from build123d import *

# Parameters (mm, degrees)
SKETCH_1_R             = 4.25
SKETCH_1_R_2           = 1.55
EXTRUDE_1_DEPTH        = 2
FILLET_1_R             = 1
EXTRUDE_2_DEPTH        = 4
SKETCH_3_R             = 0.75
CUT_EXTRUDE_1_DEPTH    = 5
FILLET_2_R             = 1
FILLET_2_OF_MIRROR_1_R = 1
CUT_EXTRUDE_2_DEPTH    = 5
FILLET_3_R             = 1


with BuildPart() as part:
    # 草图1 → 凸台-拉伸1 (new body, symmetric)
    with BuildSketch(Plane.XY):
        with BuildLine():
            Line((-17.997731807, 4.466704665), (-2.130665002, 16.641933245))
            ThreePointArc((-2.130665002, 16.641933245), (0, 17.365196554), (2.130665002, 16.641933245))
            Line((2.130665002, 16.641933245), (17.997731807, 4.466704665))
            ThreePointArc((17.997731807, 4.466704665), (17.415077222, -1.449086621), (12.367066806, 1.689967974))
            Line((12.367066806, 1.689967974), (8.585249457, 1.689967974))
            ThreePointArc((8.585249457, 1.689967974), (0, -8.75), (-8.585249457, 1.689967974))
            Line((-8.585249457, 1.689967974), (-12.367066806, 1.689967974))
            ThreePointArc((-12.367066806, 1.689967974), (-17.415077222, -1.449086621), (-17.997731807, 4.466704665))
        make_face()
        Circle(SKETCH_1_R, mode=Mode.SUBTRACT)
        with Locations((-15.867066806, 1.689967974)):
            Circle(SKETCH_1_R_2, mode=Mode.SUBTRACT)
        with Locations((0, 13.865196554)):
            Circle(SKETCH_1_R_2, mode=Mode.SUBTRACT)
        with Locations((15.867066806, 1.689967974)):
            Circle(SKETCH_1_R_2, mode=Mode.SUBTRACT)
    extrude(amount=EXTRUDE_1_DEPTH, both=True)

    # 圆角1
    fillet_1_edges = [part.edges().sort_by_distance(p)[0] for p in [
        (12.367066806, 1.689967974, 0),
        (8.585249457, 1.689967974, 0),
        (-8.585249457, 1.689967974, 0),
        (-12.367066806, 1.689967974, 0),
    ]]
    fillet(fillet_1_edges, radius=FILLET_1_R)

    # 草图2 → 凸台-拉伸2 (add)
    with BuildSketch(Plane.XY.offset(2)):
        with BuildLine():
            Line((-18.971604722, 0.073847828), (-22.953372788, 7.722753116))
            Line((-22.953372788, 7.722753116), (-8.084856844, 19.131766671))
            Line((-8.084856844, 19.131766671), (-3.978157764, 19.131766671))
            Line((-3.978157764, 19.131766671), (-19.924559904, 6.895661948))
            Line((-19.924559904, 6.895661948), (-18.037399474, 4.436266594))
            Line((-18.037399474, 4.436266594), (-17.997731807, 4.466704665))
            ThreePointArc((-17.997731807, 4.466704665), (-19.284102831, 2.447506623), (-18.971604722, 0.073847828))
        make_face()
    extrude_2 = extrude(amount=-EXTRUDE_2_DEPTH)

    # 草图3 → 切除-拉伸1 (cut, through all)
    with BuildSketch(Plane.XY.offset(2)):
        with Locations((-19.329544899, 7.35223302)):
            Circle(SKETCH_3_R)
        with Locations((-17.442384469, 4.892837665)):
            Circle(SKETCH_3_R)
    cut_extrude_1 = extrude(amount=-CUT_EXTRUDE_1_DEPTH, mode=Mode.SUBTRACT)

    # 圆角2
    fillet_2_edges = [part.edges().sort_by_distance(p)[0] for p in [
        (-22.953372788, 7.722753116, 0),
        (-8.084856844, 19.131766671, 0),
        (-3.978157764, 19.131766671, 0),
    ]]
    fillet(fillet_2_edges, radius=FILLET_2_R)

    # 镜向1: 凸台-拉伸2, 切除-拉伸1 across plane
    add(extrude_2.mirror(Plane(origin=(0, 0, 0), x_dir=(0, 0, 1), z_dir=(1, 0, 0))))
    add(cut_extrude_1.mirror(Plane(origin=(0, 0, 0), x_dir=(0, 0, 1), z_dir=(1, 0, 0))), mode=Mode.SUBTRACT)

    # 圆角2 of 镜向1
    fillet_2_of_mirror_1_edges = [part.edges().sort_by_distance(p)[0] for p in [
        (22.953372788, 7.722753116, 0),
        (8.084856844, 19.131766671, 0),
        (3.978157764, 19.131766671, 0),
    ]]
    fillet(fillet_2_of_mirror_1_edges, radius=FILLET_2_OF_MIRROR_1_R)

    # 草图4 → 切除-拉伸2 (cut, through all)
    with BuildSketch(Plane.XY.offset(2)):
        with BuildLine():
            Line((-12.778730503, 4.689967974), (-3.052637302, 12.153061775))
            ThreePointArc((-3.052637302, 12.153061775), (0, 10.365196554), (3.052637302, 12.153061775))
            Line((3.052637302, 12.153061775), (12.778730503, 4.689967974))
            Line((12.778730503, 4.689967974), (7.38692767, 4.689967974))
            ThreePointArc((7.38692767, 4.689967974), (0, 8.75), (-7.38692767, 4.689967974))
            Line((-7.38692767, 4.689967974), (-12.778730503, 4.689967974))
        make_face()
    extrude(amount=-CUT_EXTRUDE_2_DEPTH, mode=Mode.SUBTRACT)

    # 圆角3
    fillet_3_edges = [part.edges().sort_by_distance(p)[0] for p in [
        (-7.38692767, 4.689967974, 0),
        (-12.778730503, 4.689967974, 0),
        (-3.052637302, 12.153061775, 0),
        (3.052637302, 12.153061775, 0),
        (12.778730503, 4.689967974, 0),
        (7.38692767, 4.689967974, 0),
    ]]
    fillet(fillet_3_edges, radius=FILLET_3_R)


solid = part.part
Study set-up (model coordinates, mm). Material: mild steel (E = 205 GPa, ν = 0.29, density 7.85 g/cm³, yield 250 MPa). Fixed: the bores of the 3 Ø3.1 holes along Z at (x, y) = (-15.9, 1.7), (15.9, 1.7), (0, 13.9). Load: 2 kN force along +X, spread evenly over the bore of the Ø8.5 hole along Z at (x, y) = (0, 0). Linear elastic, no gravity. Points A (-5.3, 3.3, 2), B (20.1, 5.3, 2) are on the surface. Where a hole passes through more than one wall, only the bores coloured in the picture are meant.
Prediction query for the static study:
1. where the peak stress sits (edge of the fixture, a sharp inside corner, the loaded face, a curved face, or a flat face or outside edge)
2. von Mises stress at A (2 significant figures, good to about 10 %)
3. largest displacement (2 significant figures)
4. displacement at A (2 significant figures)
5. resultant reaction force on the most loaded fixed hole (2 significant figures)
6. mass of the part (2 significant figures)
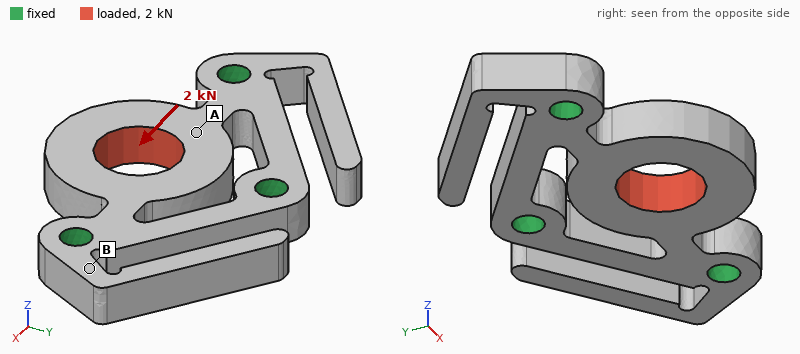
a sharp inside corner
38 MPa
9.8 µm
3.0 µm
940 N
16 g
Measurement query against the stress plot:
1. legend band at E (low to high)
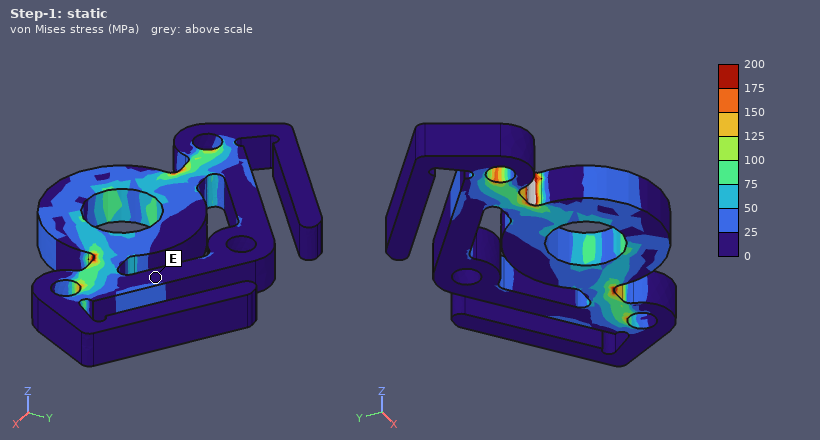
0 to 25 MPa
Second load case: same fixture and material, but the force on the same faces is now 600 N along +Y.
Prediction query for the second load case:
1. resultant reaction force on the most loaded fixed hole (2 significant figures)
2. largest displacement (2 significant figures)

320 N
5.1 µm
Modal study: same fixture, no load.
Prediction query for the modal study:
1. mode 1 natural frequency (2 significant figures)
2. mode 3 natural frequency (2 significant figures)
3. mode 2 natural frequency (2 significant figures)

3500 Hz
4500 Hz
3500 Hz
